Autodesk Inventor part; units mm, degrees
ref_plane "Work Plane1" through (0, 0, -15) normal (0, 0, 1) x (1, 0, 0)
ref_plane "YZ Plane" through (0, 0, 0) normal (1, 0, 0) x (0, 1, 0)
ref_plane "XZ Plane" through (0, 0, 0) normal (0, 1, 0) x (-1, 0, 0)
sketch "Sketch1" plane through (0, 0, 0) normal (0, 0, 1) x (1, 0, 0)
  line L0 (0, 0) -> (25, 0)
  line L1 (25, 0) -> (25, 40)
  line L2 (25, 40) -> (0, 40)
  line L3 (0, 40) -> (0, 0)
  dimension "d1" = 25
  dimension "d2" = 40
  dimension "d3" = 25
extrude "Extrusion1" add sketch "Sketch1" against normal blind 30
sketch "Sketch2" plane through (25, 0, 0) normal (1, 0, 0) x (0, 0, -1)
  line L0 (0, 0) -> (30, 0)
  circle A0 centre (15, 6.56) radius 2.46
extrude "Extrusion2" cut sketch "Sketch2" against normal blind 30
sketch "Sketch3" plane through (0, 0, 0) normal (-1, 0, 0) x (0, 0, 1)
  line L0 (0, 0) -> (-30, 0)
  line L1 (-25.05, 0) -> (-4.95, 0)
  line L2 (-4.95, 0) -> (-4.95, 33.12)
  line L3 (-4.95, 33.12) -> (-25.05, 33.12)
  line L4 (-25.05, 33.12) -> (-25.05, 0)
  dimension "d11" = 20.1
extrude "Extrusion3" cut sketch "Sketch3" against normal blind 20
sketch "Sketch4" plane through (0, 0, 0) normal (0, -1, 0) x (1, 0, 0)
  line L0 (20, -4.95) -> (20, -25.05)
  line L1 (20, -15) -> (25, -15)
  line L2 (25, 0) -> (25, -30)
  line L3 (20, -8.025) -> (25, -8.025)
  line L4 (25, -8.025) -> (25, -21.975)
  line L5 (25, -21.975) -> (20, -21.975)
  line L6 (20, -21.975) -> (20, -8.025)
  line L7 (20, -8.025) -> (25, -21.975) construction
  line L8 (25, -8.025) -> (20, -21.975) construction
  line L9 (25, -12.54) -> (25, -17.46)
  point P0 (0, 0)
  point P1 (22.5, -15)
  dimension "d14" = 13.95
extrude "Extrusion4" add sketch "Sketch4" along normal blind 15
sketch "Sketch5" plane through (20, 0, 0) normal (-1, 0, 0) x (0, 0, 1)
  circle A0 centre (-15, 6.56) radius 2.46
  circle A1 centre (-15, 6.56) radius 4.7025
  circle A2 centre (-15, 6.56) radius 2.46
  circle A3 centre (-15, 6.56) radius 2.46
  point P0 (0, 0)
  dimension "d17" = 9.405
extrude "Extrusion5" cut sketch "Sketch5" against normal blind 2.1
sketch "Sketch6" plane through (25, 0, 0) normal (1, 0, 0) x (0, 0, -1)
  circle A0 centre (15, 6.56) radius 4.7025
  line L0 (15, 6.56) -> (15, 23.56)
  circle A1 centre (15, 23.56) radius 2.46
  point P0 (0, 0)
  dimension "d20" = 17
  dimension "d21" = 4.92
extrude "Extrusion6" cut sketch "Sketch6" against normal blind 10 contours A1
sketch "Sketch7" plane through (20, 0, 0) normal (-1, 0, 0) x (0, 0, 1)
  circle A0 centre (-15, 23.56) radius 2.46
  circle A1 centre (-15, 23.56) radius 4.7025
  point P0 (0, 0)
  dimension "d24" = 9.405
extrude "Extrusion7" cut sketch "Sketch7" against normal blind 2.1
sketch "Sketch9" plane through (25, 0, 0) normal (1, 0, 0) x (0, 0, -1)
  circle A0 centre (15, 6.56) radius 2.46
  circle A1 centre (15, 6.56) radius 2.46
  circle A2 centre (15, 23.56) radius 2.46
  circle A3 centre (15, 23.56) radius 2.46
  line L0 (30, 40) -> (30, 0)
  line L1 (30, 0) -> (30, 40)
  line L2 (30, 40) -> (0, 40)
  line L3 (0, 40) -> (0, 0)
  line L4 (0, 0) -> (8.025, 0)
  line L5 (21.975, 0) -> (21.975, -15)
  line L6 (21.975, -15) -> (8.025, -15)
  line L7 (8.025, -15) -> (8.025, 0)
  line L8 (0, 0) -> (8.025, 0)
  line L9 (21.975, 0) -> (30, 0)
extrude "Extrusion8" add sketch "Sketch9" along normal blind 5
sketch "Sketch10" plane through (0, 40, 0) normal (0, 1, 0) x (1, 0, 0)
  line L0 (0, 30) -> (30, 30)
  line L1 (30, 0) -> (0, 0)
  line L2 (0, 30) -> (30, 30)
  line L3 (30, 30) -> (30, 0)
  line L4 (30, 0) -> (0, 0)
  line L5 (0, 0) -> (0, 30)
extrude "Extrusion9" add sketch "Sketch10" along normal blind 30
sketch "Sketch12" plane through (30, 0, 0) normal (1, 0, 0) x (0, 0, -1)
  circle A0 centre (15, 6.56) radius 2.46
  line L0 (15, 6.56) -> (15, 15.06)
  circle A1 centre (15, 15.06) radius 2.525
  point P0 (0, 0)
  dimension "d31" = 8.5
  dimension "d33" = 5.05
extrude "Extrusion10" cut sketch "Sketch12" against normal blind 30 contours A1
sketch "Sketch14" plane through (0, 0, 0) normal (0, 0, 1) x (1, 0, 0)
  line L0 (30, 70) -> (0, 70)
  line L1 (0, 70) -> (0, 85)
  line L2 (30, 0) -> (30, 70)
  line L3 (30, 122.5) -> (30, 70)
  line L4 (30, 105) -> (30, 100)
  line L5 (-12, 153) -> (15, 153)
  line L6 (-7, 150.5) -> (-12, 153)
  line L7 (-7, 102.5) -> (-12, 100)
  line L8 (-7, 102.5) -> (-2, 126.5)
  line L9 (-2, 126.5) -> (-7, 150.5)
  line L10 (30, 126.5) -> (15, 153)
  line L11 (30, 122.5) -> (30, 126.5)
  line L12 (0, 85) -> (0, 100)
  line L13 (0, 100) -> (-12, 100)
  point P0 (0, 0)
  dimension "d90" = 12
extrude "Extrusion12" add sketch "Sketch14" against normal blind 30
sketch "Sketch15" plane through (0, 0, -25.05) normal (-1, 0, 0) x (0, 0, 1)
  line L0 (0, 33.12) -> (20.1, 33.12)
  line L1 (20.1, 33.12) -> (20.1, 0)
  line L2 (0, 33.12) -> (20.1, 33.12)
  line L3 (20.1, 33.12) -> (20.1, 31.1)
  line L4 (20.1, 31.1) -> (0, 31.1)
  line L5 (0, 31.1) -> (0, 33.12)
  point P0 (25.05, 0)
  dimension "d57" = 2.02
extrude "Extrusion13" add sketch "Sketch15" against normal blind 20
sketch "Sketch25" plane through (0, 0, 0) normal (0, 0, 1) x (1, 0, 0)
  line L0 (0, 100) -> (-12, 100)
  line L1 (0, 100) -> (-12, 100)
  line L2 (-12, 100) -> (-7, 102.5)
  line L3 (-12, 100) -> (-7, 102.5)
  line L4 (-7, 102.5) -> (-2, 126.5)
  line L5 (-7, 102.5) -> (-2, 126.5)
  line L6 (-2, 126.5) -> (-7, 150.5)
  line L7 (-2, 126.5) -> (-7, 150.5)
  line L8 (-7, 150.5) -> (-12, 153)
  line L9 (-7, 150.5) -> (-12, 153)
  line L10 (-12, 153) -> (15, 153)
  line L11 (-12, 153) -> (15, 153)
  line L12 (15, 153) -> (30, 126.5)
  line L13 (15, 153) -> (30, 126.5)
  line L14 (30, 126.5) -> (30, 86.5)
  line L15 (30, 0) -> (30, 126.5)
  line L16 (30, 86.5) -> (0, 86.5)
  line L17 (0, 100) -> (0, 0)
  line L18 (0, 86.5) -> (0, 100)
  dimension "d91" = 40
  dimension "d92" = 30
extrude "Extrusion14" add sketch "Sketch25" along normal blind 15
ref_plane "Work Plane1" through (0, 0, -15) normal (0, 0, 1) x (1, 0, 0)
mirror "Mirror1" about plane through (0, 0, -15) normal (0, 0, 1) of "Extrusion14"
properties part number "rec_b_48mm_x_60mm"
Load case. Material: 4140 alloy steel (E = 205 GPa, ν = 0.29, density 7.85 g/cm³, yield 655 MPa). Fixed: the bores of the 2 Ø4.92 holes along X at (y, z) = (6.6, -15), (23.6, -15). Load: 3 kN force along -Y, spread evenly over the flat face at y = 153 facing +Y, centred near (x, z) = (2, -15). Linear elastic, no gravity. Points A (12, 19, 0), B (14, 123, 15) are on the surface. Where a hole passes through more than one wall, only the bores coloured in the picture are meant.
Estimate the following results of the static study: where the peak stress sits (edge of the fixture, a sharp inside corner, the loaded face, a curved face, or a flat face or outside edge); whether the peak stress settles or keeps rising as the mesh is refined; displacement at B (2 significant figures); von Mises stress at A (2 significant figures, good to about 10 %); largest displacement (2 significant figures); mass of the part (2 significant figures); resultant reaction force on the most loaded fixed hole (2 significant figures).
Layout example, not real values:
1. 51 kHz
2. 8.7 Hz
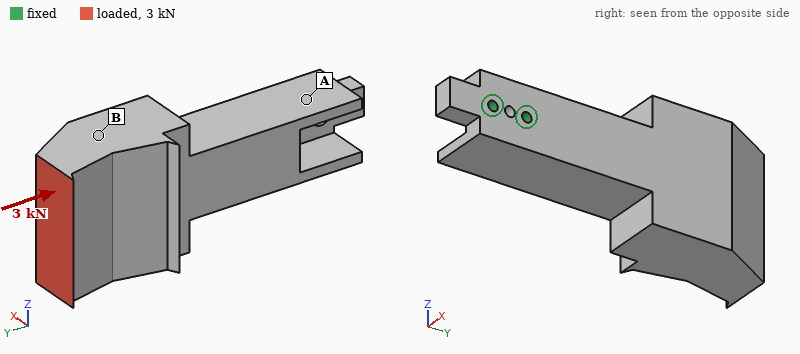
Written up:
1. edge of the fixture
2. keeps rising
3. 64 µm
4. 22 MPa
5. 92 µm
6. 1.5 kg
7. 3.4 kN
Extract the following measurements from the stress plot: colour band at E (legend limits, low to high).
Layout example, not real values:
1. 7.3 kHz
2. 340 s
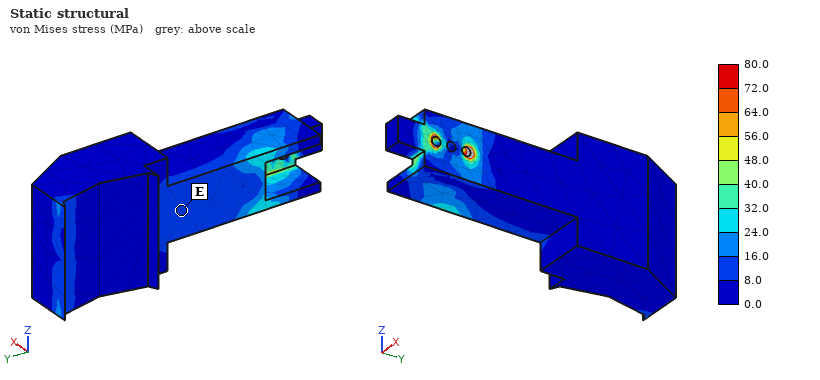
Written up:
1. 8.0 to 16.0 MPa
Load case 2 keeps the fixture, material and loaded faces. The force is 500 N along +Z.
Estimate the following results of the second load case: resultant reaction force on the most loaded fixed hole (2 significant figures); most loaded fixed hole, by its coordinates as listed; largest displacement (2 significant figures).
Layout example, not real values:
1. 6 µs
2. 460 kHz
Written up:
1. 3.3 kN
2. (23.6, -15)
3. 68 µm
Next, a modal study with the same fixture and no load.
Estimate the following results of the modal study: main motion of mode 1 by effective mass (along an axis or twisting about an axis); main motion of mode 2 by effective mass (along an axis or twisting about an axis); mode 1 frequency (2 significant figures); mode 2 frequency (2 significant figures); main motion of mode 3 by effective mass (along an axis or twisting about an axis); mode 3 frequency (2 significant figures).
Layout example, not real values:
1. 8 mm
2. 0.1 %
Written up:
1. along X
2. along Z
3. 520 Hz
4. 600 Hz
5. twisting about Y
6. 1600 Hz
